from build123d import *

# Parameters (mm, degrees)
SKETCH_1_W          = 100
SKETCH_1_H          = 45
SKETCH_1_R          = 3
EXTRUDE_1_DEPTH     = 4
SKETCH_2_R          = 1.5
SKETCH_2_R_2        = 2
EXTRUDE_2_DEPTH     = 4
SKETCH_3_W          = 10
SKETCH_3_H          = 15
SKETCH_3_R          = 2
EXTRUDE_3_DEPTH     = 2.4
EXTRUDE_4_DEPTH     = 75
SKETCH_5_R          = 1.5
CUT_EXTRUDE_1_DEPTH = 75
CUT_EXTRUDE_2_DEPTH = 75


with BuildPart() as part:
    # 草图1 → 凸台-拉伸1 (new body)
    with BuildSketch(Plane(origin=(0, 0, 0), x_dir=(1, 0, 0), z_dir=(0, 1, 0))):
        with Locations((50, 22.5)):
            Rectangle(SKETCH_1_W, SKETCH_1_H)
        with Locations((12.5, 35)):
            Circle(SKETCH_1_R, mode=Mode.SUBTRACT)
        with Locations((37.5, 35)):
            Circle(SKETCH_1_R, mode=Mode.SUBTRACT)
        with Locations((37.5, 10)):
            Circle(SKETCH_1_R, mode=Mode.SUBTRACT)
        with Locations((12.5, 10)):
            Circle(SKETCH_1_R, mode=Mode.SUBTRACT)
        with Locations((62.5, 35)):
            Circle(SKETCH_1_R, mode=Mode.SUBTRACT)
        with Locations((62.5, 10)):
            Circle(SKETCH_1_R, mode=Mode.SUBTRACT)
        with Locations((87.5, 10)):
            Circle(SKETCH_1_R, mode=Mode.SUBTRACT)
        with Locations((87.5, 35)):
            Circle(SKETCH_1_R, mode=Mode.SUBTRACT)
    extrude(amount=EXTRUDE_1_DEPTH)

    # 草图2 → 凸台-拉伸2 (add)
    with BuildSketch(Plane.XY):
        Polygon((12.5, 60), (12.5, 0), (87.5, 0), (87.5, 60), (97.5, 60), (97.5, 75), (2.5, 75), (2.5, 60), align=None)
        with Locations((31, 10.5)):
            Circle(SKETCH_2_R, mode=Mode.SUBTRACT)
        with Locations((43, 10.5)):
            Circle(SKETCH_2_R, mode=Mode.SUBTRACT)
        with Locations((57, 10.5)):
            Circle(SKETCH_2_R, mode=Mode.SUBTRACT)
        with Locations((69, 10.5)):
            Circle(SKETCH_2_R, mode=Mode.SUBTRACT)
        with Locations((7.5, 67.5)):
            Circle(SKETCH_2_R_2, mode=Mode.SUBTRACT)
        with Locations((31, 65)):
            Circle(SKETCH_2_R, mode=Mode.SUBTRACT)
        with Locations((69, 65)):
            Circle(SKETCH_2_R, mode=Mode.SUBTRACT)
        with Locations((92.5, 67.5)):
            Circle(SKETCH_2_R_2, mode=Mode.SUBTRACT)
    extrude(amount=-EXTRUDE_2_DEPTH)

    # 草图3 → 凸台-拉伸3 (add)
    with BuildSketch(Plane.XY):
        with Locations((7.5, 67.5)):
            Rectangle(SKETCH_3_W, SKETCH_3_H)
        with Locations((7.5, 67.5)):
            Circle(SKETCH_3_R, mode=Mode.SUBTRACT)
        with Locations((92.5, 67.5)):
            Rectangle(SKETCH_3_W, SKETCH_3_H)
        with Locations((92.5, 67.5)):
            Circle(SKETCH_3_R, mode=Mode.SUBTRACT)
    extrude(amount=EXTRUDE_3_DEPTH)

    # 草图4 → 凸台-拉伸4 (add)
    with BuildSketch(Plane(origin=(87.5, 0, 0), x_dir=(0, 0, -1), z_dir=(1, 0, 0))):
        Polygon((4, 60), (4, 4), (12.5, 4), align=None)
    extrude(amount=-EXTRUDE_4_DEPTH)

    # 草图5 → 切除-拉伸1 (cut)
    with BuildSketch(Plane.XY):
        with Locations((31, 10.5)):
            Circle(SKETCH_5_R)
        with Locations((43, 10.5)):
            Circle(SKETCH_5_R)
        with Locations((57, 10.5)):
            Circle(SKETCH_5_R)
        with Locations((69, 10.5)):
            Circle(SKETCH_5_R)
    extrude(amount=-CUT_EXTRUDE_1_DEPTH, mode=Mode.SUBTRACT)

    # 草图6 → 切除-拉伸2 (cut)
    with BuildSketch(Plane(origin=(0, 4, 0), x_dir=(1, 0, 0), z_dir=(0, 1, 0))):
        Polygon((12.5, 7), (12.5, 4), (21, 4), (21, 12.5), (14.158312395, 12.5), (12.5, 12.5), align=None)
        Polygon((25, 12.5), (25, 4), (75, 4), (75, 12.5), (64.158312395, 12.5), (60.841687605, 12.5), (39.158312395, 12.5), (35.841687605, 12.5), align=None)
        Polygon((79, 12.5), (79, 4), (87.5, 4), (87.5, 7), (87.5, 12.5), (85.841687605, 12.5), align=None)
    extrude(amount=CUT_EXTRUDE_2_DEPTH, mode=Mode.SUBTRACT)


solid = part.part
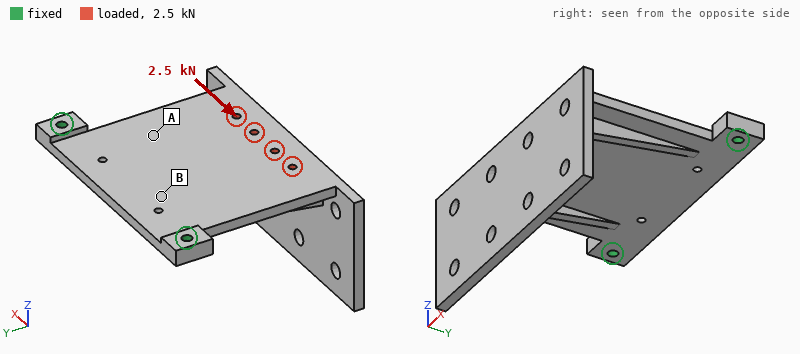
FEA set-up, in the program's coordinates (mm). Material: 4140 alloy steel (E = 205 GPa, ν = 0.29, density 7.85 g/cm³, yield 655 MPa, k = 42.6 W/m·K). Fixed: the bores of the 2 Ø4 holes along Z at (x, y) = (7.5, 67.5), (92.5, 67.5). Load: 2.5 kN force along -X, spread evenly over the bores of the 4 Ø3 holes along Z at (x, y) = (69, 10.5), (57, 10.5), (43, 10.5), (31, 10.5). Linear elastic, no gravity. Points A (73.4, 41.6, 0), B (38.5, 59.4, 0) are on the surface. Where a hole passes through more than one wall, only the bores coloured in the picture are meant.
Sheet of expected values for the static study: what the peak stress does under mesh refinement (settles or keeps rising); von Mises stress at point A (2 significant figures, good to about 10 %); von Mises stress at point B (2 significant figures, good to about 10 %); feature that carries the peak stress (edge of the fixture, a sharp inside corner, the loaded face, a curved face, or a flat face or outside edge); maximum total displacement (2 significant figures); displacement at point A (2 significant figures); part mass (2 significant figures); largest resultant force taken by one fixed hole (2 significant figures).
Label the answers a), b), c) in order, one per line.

a) keeps rising
b) 22 MPa
c) 8.8 MPa
d) edge of the fixture
e) 25 µm
f) 8.5 µm
g) 330 g
h) 2.2 kN
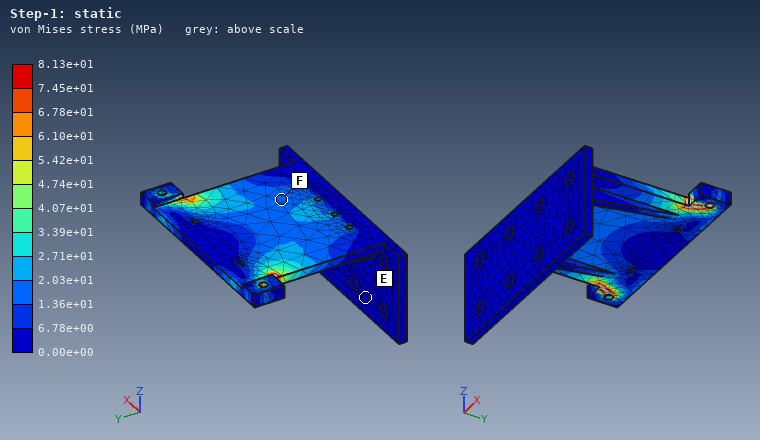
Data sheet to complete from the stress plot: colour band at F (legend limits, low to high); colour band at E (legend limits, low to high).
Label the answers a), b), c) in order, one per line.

a) 1.36e+01 to 2.03e+01 MPa
b) 0.00e+00 to 6.78e+00 MPa
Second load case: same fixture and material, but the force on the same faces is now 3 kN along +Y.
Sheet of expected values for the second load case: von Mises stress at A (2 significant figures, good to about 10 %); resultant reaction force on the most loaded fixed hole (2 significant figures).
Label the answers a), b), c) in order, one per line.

a) 17 MPa
b) 1.7 kN
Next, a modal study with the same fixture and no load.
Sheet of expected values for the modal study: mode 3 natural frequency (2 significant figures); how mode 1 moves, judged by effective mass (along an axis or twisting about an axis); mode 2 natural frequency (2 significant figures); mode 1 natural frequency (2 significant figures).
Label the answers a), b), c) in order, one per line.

a) 1600 Hz
b) along Z
c) 680 Hz
d) 280 Hz
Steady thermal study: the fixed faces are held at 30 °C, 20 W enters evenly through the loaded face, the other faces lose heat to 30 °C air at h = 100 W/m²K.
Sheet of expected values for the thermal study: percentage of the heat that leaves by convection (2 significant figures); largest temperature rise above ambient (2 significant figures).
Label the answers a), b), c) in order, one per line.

a) 94 %
b) 28 K
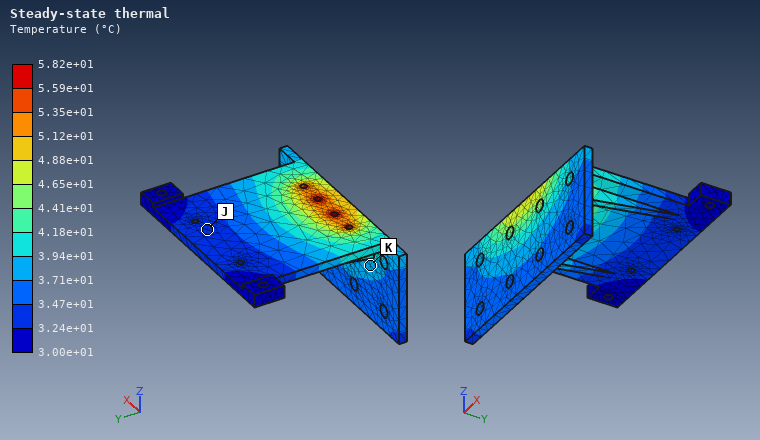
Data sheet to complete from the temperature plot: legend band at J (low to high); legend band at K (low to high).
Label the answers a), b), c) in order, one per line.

a) 3.24e+01 to 3.47e+01 °C
b) 3.71e+01 to 3.94e+01 °C
